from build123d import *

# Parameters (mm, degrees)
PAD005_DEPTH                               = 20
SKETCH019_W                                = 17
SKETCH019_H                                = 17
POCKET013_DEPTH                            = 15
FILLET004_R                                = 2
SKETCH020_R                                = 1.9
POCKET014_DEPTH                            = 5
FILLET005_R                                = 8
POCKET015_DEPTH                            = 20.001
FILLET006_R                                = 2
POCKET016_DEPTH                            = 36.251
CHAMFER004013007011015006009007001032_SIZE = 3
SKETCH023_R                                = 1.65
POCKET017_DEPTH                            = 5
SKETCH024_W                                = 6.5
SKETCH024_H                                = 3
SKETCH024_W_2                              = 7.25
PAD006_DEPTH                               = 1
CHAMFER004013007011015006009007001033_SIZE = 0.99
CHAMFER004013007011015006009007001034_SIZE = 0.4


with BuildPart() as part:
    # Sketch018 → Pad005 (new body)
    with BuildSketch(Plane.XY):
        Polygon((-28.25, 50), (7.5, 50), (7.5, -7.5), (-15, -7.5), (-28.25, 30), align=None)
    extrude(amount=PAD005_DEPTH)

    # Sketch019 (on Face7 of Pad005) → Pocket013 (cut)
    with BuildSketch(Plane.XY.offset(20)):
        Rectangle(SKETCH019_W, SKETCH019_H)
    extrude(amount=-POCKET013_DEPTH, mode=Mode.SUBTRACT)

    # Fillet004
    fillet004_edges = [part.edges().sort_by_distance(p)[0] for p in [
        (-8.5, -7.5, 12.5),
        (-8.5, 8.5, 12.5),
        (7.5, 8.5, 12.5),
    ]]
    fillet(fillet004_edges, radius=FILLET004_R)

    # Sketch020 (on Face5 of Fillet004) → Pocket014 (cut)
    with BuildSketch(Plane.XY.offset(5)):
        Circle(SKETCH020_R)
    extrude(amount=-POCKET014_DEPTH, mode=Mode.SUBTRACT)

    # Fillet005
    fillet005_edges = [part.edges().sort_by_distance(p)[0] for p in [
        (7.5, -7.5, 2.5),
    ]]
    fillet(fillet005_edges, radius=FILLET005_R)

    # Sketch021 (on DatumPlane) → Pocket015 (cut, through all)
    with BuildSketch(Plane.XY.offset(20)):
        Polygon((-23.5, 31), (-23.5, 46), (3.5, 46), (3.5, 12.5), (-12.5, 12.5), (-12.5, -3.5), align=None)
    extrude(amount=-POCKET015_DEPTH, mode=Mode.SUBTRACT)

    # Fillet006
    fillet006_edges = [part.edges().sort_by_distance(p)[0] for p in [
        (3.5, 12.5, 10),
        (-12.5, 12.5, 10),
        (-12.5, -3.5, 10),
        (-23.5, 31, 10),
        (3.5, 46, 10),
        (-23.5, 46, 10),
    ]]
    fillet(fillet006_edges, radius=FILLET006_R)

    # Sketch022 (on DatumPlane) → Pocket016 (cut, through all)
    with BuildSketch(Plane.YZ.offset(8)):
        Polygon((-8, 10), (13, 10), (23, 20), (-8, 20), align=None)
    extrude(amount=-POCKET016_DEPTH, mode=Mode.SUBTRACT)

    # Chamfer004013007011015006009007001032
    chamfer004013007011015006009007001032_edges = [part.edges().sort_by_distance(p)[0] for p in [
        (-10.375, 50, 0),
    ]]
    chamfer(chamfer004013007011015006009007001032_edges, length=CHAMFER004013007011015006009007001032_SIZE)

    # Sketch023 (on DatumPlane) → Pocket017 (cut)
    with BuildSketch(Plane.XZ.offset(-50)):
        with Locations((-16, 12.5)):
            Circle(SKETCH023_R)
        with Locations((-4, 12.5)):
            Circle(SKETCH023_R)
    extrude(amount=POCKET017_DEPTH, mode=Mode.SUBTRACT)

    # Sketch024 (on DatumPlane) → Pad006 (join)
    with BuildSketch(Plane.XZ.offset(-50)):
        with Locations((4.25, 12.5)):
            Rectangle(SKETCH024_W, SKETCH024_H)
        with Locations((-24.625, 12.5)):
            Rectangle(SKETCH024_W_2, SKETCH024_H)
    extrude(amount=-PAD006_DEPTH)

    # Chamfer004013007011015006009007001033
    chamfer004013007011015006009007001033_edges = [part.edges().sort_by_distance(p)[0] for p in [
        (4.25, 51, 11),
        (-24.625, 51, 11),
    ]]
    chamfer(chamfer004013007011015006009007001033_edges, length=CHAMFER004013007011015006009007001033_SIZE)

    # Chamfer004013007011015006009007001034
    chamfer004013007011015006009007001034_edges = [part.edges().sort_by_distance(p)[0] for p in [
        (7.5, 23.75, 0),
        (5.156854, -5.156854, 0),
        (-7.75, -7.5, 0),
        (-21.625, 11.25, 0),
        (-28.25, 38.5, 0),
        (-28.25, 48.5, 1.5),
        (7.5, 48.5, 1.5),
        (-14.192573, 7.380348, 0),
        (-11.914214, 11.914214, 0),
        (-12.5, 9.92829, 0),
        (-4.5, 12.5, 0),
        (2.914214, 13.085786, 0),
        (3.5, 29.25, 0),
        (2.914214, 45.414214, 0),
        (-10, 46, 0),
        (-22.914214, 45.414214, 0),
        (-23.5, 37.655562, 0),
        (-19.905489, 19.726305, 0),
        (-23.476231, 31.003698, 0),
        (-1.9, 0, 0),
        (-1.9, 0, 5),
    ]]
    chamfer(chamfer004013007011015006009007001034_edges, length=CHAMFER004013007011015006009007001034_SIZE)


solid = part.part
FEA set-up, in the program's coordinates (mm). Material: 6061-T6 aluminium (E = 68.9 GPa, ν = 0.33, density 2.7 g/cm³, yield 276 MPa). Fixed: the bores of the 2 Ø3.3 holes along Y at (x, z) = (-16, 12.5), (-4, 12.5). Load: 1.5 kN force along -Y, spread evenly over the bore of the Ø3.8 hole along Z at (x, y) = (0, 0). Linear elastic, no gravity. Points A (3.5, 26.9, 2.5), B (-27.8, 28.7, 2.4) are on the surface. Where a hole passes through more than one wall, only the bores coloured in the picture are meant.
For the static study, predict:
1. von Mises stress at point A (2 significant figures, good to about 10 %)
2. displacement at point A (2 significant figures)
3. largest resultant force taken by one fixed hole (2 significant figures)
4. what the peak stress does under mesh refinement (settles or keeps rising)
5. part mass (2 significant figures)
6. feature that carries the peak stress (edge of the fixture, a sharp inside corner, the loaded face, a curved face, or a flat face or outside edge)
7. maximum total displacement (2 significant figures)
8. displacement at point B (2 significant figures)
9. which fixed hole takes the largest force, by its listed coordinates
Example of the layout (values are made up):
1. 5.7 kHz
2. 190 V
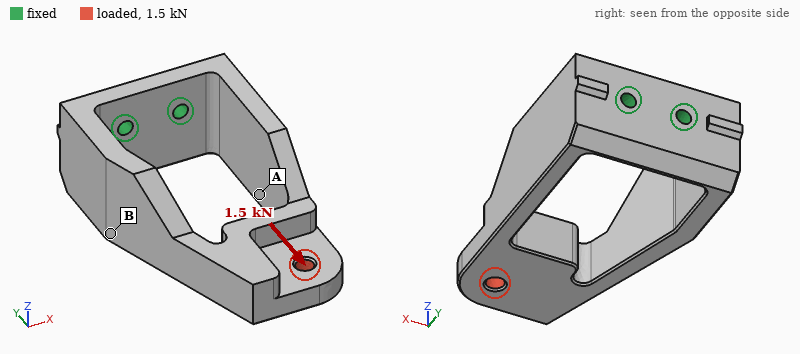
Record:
1. 60 MPa
2. 0.20 mm
3. 1.4 kN
4. keeps rising
5. 31 g
6. edge of the fixture
7. 0.43 mm
8. 0.10 mm
9. (-4, 12.5)
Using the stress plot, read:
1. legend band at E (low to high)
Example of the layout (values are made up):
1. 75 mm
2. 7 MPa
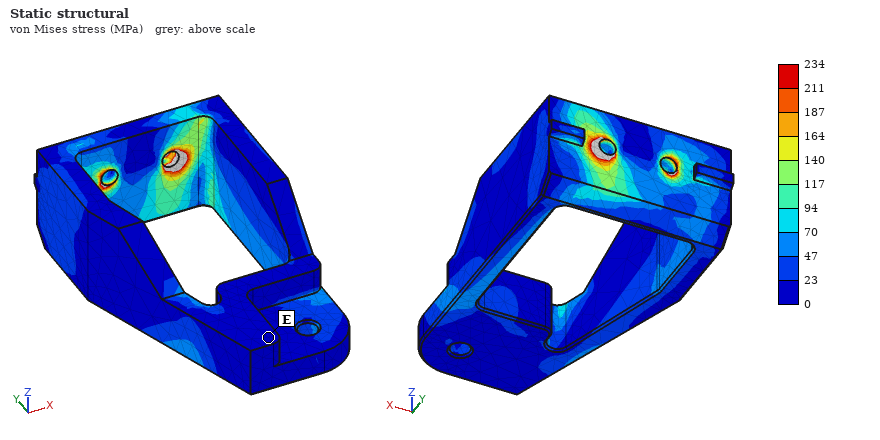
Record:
1. 0 to 23 MPa
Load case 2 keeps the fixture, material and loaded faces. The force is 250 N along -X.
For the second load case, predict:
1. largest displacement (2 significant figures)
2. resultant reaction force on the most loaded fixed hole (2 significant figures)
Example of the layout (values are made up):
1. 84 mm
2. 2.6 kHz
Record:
1. 0.21 mm
2. 530 N
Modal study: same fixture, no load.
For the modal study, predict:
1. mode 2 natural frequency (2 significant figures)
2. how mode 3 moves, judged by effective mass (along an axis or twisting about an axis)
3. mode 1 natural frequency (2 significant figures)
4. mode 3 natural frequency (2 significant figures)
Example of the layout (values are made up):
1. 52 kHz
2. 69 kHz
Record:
1. 1500 Hz
2. twisting about Y
3. 1500 Hz
4. 4500 Hz
